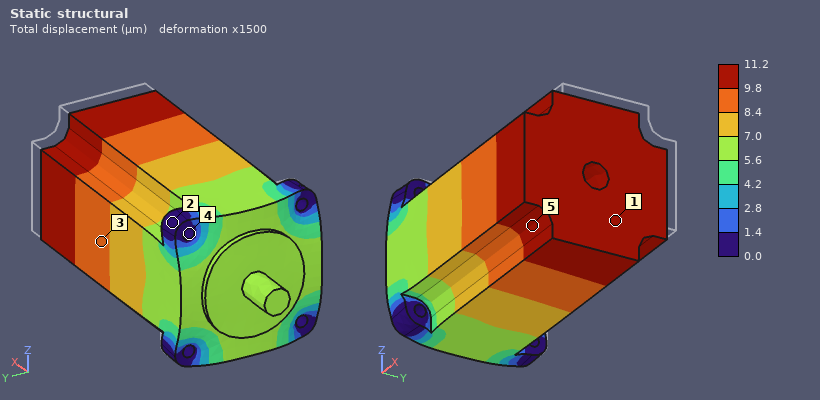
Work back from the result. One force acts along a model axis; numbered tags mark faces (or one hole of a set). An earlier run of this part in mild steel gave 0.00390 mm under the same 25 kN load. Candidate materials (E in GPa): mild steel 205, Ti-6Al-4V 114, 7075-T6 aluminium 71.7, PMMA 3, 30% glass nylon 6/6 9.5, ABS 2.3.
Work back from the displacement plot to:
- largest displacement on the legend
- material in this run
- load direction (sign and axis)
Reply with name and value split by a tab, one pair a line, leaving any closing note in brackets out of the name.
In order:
largest displacement on the legend	11.2 µm
material in this run	7075-T6 aluminium
load direction	-X
